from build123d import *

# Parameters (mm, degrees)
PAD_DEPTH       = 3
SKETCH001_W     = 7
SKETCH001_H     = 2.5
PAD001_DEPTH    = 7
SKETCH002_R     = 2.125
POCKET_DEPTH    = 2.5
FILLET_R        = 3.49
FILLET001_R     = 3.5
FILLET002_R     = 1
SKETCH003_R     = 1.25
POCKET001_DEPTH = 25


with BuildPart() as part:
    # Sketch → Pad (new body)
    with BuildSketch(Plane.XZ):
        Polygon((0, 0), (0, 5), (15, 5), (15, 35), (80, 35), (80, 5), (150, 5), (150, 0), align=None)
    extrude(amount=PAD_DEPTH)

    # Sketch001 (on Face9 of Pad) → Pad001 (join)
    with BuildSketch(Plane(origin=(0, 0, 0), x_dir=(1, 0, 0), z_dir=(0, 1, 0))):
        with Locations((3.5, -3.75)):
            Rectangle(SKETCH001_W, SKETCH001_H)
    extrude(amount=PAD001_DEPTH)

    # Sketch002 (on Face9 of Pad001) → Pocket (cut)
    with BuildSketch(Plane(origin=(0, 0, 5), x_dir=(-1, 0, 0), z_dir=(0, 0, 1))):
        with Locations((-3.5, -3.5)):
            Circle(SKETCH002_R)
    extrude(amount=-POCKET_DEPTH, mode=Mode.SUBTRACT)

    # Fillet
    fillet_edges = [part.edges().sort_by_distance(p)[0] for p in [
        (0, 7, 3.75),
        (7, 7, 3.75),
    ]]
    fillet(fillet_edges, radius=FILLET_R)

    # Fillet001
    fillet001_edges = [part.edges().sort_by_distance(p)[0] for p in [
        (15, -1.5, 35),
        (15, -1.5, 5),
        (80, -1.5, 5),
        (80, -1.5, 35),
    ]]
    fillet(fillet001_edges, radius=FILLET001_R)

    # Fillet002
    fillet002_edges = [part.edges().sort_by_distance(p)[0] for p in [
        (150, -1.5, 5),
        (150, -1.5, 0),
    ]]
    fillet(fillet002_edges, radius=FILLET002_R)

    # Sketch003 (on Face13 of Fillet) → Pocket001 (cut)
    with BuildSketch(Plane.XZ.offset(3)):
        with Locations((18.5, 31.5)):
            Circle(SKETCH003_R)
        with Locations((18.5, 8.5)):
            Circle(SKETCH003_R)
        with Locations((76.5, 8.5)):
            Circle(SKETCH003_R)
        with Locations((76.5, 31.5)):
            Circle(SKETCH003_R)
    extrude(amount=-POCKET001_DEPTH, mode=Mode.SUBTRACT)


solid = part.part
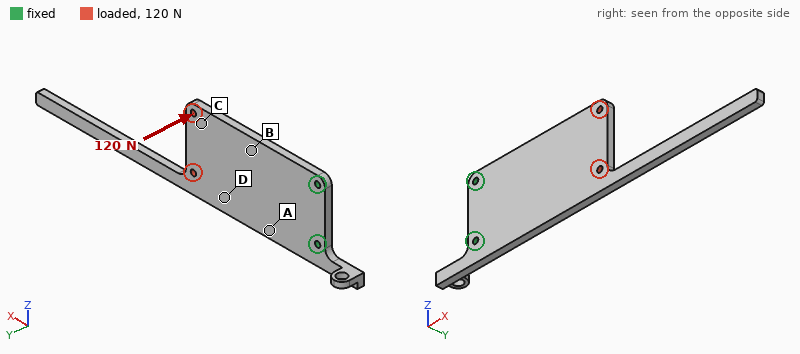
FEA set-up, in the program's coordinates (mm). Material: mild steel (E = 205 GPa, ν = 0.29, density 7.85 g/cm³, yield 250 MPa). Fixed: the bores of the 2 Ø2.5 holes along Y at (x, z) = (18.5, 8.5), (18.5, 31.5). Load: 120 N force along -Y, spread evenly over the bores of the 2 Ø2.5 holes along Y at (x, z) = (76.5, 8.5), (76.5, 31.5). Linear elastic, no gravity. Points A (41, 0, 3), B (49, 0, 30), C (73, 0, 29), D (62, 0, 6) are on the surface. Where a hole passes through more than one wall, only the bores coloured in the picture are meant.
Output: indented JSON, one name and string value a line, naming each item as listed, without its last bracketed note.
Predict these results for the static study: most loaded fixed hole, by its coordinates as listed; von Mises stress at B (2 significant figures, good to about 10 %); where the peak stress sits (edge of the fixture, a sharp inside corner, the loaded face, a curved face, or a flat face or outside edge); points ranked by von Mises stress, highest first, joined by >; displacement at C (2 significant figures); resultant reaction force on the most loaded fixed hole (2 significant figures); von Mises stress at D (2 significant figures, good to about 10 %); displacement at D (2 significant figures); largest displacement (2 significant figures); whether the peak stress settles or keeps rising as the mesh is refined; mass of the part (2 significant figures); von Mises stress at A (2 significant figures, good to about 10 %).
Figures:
{
  "most loaded fixed hole, by its coordinates as listed": "(18.5, 8.5)",
  "von Mises stress at B": "64 MPa",
  "where the peak stress sits": "edge of the fixture",
  "points ranked by von Mises stress, highest first, joined by >": "A > B > D > C",
  "displacement at C": "0.48 mm",
  "resultant reaction force on the most loaded fixed hole": "71 N",
  "von Mises stress at D": "34 MPa",
  "displacement at D": "0.33 mm",
  "largest displacement": "1.5 mm",
  "whether the peak stress settles or keeps rising as the mesh is refined": "keeps rising",
  "mass of the part": "64 g",
  "von Mises stress at A": "81 MPa"
}
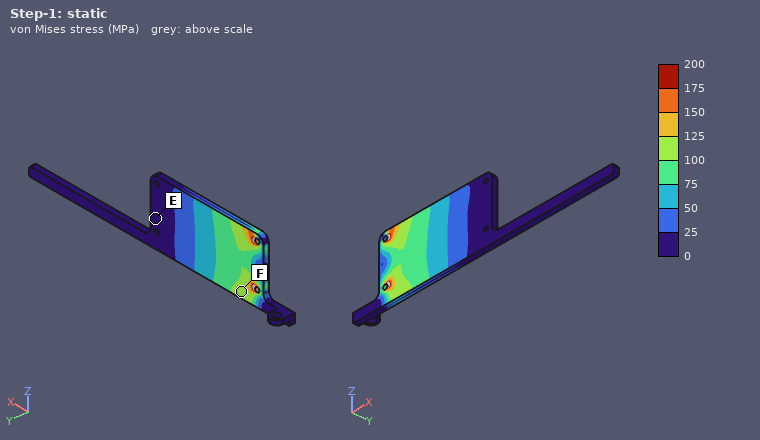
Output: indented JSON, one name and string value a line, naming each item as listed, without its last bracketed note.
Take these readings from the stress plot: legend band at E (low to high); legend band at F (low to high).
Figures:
{
  "legend band at E": "0 to 25 MPa",
  "legend band at F": "100 to 125 MPa"
}
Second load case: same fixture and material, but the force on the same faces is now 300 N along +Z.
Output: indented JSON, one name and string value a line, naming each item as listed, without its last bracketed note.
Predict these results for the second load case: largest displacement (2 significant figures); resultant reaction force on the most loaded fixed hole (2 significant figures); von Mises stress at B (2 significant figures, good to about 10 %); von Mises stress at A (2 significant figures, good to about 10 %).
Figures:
{
  "largest displacement": "36 µm",
  "resultant reaction force on the most loaded fixed hole": "750 N",
  "von Mises stress at B": "10 MPa",
  "von Mises stress at A": "14 MPa"
}
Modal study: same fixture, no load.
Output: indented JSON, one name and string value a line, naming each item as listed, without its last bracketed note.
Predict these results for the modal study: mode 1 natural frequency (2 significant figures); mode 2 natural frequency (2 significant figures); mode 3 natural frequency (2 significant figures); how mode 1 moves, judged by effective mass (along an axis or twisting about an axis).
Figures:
{
  "mode 1 natural frequency": "280 Hz",
  "mode 2 natural frequency": "800 Hz",
  "mode 3 natural frequency": "800 Hz",
  "how mode 1 moves, judged by effective mass": "along Y"
}
